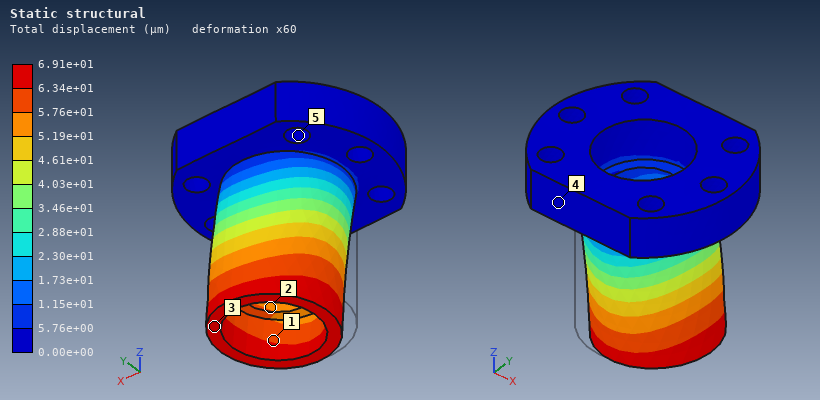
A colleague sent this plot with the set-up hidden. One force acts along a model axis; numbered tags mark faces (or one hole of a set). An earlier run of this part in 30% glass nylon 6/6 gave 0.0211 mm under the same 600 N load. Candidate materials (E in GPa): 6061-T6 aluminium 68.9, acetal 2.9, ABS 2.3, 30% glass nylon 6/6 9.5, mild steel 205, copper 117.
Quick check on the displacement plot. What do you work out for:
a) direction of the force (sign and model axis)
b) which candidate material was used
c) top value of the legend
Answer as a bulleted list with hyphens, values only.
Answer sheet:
- +X
- acetal
- 6.91e+01 µm
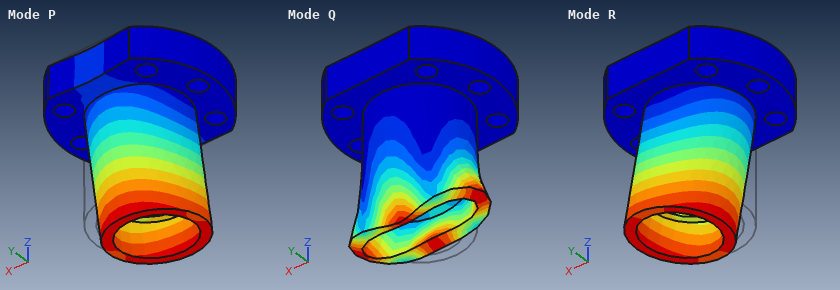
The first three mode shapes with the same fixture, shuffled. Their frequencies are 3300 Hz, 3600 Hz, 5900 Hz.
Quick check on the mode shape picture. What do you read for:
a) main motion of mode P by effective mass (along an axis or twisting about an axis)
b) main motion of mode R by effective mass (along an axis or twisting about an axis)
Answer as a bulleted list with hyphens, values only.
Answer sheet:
- along Y
- along X
